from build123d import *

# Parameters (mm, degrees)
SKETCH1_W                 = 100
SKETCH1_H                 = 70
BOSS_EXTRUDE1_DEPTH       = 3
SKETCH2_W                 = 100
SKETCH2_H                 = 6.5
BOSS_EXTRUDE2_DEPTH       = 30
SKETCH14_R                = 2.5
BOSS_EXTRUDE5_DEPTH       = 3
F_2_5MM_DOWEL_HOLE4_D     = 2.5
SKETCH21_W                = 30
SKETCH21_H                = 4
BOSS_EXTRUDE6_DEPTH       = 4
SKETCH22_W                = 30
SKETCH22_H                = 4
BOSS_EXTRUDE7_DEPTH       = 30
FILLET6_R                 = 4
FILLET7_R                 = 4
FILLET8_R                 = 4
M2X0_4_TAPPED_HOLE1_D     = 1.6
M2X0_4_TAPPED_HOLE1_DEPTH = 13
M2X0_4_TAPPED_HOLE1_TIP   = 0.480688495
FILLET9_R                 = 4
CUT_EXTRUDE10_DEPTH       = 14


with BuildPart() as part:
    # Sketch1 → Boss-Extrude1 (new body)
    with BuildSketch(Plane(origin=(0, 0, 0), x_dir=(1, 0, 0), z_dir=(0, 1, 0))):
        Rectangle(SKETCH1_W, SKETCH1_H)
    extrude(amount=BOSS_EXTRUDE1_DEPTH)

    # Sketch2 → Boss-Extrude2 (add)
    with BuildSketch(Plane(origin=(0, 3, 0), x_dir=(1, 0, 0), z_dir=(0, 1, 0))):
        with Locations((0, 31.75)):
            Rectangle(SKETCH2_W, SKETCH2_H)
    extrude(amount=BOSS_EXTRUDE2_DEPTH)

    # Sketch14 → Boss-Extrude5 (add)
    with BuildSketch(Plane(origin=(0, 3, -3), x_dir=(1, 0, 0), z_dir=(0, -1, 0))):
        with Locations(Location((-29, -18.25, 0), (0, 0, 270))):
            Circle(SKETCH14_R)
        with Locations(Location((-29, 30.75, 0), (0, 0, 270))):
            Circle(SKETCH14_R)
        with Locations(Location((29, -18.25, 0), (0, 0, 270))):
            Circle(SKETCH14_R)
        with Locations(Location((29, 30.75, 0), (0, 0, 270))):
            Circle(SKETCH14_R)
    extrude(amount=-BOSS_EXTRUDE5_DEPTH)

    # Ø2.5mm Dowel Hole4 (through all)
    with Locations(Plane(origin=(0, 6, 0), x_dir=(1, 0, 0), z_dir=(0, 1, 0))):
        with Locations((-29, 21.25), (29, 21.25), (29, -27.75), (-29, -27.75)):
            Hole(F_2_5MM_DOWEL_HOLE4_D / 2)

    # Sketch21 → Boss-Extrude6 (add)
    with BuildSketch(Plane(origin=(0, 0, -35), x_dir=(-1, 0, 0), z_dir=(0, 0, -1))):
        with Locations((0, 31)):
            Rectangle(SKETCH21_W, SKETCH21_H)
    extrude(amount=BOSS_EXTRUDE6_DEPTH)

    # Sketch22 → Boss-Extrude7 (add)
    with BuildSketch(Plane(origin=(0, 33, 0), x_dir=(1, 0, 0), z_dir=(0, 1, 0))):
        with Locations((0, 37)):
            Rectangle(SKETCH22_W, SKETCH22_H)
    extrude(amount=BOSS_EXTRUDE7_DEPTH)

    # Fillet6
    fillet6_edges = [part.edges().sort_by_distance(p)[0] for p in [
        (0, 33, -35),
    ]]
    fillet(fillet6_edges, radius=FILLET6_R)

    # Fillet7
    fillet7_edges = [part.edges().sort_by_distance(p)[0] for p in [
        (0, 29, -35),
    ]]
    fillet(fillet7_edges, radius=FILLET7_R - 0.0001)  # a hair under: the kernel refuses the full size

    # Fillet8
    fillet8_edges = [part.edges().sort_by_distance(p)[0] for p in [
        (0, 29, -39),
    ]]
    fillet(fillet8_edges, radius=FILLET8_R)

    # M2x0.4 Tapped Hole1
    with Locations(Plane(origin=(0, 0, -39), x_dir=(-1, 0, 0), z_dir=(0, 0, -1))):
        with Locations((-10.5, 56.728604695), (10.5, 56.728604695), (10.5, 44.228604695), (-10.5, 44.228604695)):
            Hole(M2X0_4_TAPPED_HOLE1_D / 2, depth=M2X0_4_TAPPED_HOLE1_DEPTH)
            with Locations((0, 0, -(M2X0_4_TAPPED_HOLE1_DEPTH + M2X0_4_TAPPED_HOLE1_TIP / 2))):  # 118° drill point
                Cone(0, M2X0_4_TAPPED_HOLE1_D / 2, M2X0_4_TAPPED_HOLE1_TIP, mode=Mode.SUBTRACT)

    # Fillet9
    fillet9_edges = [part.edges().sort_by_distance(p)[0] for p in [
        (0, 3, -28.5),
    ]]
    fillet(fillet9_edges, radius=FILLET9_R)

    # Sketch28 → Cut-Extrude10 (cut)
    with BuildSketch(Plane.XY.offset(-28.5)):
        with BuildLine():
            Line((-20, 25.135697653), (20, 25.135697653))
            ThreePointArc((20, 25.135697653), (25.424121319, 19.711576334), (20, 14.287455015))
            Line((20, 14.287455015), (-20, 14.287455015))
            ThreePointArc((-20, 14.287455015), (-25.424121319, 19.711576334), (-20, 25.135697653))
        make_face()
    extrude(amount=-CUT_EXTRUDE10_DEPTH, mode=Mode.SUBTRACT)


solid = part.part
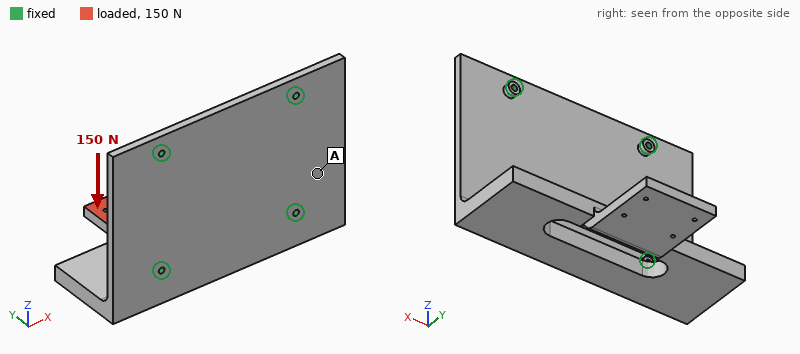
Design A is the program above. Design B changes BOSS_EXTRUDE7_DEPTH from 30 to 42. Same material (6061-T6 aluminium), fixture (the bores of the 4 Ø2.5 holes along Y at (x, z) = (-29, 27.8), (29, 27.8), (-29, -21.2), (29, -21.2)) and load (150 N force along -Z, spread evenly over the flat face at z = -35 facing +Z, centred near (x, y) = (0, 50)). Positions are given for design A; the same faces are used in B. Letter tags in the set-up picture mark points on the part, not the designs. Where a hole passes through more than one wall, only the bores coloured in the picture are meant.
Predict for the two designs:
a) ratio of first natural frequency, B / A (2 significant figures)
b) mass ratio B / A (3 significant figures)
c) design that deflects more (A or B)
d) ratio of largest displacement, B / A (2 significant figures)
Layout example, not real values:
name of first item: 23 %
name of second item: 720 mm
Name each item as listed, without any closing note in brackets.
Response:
ratio of first natural frequency, B / A: 0.77
mass ratio B / A: 1.03
design that deflects more: B
ratio of largest displacement, B / A: 1.5
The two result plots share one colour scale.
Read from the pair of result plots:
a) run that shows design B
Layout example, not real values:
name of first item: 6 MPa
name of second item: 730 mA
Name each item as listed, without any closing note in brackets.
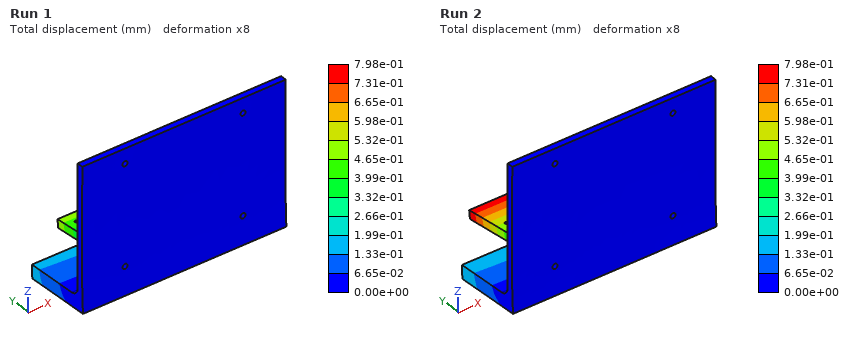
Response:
run that shows design B: Run 2
